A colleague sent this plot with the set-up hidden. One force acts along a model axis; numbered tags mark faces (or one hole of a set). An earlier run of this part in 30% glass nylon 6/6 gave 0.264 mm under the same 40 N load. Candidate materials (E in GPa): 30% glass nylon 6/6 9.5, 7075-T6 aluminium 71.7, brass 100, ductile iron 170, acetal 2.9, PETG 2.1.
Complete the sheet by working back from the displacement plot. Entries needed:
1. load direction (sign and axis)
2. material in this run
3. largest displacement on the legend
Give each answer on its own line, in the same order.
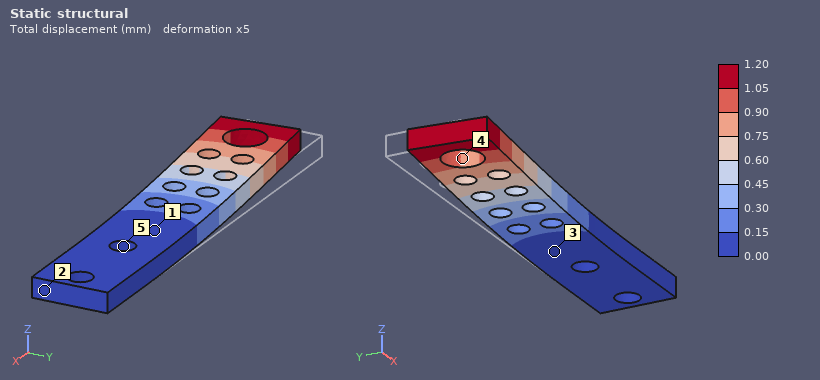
-Y
PETG
1.20 mm
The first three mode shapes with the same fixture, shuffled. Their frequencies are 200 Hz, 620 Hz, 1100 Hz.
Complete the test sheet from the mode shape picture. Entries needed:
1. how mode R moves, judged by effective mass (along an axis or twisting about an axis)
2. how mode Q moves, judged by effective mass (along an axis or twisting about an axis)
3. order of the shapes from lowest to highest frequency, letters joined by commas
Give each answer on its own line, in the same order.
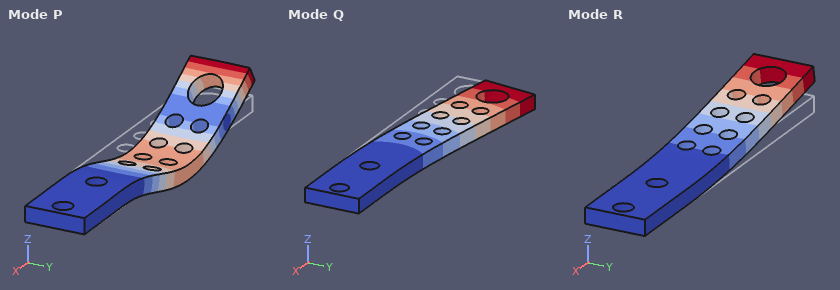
along Z
along Y
R, Q, P
